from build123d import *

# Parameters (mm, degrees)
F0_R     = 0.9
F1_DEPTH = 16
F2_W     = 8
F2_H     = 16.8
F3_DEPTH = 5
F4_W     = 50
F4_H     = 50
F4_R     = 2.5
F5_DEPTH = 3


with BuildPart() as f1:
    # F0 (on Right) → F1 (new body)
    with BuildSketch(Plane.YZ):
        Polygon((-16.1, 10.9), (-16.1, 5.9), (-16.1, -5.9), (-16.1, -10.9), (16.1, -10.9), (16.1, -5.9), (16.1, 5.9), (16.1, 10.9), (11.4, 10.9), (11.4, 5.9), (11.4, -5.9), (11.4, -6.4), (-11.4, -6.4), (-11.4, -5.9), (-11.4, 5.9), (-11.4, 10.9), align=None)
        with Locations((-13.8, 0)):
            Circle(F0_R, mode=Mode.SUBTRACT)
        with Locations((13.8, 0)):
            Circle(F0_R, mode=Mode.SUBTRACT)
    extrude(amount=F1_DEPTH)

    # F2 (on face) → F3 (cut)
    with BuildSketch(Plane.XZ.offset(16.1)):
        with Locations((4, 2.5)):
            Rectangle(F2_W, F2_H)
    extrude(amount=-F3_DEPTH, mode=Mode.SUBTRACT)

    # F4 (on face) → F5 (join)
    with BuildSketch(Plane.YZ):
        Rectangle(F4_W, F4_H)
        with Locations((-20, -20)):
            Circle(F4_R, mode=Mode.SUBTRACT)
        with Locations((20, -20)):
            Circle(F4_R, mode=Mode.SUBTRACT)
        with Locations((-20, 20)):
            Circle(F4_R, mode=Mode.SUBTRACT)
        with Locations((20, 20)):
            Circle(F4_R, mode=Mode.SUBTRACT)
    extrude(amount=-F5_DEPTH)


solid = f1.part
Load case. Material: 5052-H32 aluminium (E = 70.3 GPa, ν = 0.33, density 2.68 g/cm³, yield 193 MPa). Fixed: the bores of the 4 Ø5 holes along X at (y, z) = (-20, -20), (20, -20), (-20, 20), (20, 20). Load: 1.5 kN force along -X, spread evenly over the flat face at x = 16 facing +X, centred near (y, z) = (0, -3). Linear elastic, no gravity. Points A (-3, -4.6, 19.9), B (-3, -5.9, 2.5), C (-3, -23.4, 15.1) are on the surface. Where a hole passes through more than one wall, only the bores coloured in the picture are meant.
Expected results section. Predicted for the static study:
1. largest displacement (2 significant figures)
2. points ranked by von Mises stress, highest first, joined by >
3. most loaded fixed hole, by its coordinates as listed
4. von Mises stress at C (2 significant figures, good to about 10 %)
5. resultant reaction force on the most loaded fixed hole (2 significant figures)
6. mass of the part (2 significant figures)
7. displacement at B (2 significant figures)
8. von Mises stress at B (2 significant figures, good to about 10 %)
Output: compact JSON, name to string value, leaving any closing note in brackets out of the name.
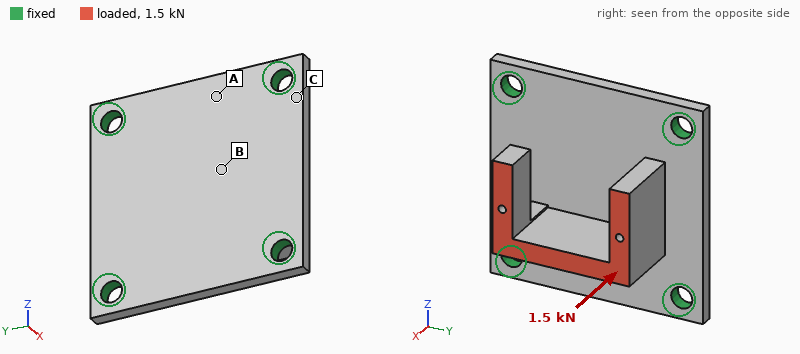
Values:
{"largest displacement": "0.23 mm", "points ranked by von Mises stress, highest first, joined by >": "C > B > A", "most loaded fixed hole, by its coordinates as listed": "(-20, -20)", "von Mises stress at C": "45 MPa", "resultant reaction force on the most loaded fixed hole": "560 N", "mass of the part": "31 g", "displacement at B": "0.046 mm", "von Mises stress at B": "30 MPa"}
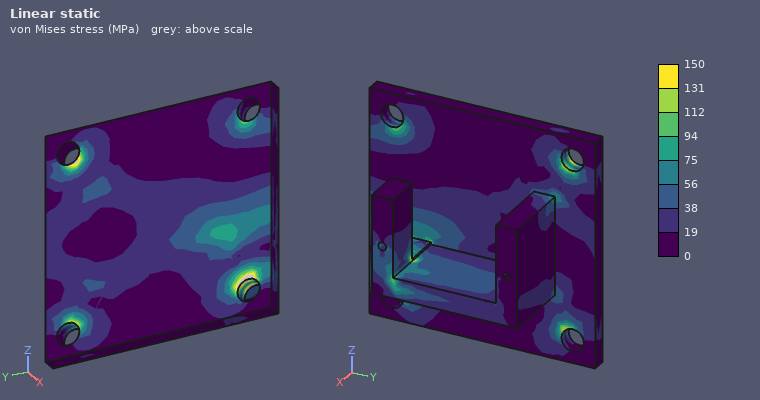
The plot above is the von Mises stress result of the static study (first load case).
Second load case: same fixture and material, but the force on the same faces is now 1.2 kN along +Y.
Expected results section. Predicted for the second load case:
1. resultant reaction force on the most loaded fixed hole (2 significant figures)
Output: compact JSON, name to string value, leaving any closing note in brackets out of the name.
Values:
{"resultant reaction force on the most loaded fixed hole": "670 N"}
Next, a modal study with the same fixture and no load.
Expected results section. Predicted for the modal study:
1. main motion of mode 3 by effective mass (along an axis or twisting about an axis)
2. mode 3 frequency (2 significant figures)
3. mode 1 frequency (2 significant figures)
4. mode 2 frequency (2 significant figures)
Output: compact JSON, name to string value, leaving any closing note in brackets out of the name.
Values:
{"main motion of mode 3 by effective mass": "along X", "mode 3 frequency": "8100 Hz", "mode 1 frequency": "5100 Hz", "mode 2 frequency": "7100 Hz"}
